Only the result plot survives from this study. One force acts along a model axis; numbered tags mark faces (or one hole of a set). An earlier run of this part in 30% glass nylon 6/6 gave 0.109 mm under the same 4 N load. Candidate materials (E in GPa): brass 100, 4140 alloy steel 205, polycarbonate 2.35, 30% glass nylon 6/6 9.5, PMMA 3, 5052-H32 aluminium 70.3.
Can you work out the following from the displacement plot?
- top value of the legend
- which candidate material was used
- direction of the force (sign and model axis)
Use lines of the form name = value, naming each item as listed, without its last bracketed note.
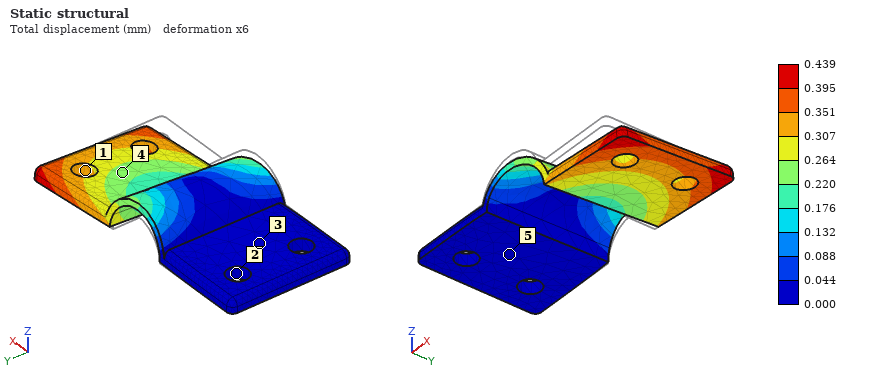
top value of the legend = 0.439 mm
which candidate material was used = polycarbonate
direction of the force = +Y
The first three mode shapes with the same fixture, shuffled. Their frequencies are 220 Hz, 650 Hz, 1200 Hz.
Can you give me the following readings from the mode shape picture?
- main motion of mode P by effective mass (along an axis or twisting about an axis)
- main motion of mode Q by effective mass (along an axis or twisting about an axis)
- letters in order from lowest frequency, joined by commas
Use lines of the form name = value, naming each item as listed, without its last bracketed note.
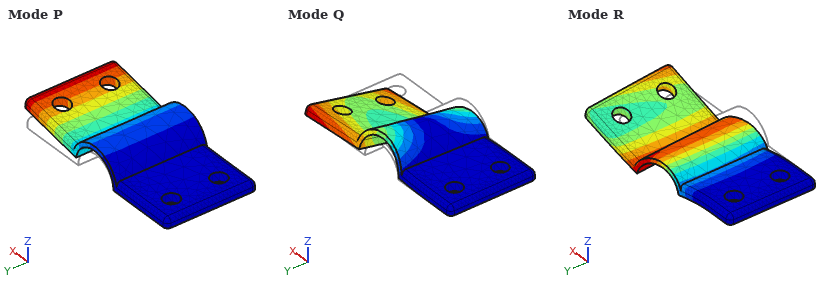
main motion of mode P by effective mass = along Z
main motion of mode Q by effective mass = along Y
letters in order from lowest frequency, joined by commas = P, Q, R
